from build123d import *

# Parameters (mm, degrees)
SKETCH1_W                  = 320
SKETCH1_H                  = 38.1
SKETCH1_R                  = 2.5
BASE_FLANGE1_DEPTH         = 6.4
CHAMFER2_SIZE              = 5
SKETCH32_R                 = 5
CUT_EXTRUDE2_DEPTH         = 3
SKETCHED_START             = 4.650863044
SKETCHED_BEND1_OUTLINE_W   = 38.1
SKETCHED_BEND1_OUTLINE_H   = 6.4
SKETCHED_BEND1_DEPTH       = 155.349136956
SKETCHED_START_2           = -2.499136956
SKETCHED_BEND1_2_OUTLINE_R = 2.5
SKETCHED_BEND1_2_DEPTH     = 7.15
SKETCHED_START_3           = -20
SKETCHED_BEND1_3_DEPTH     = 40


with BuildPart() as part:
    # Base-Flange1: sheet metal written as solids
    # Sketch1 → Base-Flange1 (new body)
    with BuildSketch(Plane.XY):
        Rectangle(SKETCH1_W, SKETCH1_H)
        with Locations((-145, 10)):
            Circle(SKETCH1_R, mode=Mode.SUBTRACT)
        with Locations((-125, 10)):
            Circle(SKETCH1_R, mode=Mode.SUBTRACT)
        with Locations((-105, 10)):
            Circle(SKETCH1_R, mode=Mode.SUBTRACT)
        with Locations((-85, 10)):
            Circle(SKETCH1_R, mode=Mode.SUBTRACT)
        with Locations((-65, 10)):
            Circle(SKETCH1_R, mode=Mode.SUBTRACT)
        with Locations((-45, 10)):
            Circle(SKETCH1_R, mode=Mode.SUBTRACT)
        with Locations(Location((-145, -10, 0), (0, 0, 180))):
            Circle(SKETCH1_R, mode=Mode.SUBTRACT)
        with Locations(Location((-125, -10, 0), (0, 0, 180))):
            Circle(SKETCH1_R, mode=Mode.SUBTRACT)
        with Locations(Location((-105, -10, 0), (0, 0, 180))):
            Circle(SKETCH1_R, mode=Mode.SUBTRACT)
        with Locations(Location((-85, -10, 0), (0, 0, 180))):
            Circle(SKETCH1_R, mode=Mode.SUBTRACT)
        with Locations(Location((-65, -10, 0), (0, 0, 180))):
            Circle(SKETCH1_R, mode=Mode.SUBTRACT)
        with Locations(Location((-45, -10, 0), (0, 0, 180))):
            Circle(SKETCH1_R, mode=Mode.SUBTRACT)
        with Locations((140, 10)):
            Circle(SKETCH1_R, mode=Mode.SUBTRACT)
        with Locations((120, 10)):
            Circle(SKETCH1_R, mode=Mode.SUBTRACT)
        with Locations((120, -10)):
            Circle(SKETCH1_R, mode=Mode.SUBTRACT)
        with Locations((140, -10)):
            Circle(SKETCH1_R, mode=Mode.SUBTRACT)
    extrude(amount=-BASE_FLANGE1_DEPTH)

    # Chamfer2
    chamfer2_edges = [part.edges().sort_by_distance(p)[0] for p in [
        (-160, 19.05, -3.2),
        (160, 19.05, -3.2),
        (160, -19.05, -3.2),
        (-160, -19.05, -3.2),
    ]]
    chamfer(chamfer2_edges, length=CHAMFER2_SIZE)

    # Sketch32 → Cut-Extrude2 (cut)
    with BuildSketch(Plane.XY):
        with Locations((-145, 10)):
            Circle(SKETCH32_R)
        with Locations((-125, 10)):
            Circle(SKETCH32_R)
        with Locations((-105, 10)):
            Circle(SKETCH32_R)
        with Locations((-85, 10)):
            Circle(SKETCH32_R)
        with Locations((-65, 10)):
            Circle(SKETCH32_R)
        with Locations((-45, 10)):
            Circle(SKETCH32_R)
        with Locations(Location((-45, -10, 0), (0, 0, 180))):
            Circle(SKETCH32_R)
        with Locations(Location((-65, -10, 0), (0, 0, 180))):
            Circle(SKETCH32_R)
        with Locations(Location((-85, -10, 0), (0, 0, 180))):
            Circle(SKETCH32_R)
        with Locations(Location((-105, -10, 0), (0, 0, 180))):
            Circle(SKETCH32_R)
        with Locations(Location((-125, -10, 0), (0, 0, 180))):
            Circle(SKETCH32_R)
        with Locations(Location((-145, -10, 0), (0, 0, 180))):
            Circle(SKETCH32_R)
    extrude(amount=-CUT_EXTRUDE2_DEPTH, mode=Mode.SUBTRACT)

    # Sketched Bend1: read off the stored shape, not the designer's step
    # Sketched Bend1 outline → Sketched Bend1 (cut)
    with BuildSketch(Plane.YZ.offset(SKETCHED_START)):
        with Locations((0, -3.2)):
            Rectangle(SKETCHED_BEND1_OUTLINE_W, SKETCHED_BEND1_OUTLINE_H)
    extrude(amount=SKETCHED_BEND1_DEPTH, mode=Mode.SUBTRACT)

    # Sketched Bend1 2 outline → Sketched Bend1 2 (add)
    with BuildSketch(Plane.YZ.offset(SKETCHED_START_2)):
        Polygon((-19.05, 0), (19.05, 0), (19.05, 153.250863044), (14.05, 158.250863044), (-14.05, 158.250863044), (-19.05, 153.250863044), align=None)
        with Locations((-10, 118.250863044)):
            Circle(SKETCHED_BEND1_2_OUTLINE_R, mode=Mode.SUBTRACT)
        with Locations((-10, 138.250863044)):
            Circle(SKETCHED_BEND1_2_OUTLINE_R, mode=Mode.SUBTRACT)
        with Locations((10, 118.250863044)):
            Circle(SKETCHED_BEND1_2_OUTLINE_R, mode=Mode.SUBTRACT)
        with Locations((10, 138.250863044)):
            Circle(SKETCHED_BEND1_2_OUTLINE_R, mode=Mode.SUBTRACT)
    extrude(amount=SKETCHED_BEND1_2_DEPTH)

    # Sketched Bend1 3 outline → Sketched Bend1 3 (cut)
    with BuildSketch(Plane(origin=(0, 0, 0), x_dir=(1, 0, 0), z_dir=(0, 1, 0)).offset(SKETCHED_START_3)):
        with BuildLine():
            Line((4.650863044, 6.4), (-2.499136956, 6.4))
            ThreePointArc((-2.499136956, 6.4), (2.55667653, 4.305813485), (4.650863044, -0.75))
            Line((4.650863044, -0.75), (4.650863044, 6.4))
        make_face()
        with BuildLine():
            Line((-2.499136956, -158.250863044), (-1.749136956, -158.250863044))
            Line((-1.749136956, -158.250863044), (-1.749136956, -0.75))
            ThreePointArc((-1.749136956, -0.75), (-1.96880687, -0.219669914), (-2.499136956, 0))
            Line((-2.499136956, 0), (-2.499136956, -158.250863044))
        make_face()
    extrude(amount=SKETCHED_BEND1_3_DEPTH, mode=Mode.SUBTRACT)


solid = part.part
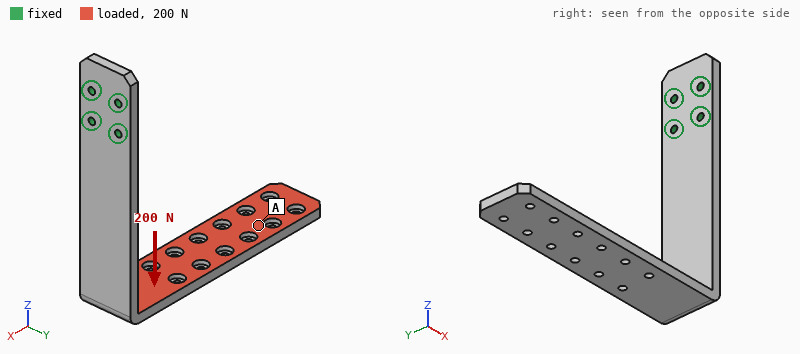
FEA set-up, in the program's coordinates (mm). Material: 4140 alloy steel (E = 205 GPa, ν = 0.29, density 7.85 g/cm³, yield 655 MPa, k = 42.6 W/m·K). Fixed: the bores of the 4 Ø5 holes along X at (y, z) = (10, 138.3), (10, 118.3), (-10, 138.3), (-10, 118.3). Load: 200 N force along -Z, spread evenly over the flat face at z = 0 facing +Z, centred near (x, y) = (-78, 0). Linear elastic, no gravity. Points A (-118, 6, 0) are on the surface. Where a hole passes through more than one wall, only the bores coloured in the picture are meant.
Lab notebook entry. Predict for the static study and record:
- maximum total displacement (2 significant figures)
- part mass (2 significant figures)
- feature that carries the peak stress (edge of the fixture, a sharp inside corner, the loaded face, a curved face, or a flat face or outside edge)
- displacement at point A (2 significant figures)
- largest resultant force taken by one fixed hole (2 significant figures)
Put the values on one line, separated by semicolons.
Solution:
2.6 mm; 580 g; a curved face; 1.9 mm; 120 N
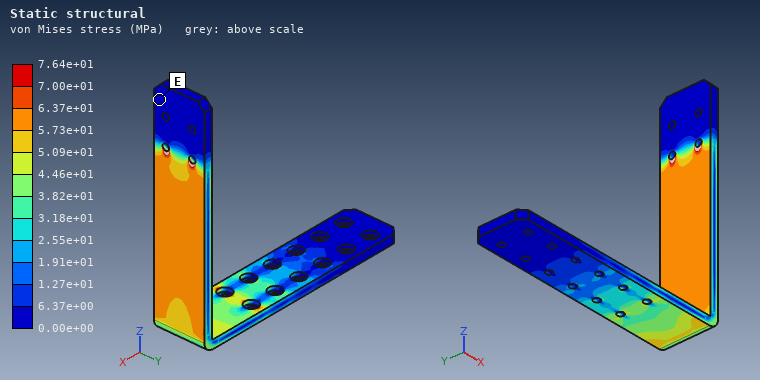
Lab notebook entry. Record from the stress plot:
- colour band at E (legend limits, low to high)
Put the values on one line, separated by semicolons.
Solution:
0.00e+00 to 6.37e+00 MPa
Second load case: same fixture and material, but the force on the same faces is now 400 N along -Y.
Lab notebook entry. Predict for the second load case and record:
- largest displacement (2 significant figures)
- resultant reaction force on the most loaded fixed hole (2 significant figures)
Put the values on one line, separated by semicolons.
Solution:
2.4 mm; 2.1 kN
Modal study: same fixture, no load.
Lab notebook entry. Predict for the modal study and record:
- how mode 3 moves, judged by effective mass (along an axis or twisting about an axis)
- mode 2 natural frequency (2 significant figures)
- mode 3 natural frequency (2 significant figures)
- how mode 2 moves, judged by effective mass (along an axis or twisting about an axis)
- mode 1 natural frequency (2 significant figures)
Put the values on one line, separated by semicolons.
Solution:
along X; 150 Hz; 250 Hz; along Y; 92 Hz
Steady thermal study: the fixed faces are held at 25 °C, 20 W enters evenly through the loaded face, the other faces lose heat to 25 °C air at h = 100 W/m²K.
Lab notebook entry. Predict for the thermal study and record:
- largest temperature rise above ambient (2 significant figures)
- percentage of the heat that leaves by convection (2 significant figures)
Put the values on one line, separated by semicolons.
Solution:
18 K; 99 %
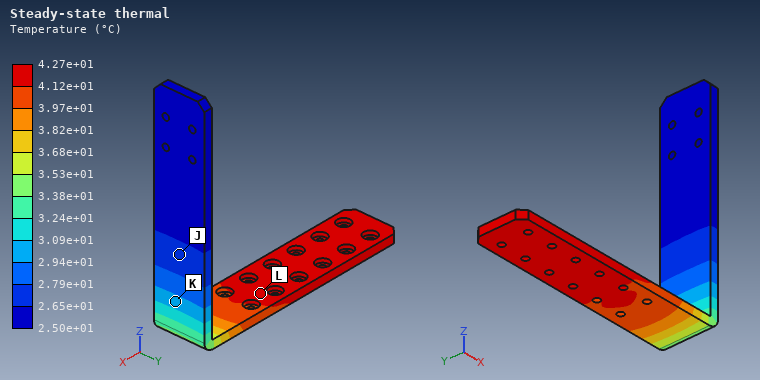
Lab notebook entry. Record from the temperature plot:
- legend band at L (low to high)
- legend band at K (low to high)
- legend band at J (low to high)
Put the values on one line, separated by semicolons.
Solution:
4.12e+01 to 4.27e+01 °C; 2.94e+01 to 3.09e+01 °C; 2.65e+01 to 2.79e+01 °C
